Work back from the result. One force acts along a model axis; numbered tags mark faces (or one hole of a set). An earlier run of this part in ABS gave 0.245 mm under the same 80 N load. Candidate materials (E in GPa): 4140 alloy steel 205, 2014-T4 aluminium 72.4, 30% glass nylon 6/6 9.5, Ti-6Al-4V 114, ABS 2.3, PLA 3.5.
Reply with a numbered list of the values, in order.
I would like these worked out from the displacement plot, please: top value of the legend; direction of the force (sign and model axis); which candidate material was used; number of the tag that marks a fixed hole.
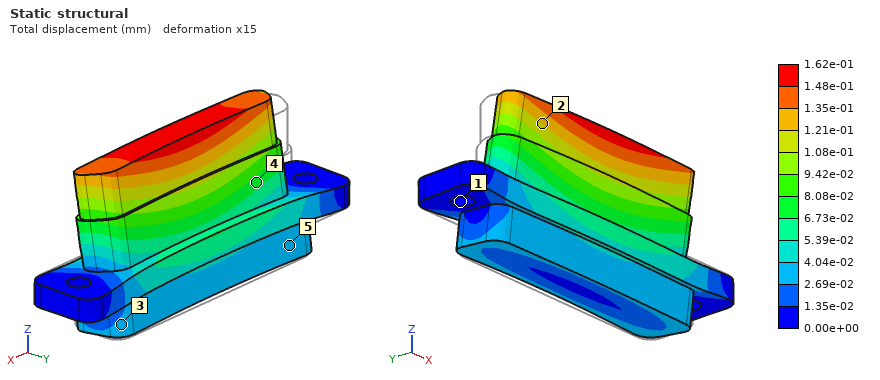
1. 1.62e-01 mm
2. -Y
3. PLA
4. 1
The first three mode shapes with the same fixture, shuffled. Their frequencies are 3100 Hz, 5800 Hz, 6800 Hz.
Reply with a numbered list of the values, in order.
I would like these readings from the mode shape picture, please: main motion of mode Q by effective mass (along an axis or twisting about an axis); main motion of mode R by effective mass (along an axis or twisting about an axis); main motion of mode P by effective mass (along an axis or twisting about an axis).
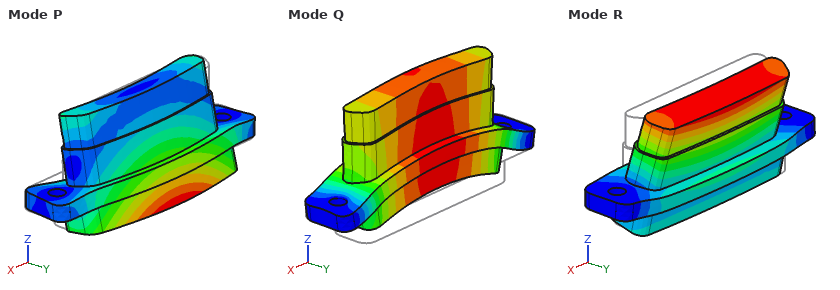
1. along Z
2. along Y
3. along Y
